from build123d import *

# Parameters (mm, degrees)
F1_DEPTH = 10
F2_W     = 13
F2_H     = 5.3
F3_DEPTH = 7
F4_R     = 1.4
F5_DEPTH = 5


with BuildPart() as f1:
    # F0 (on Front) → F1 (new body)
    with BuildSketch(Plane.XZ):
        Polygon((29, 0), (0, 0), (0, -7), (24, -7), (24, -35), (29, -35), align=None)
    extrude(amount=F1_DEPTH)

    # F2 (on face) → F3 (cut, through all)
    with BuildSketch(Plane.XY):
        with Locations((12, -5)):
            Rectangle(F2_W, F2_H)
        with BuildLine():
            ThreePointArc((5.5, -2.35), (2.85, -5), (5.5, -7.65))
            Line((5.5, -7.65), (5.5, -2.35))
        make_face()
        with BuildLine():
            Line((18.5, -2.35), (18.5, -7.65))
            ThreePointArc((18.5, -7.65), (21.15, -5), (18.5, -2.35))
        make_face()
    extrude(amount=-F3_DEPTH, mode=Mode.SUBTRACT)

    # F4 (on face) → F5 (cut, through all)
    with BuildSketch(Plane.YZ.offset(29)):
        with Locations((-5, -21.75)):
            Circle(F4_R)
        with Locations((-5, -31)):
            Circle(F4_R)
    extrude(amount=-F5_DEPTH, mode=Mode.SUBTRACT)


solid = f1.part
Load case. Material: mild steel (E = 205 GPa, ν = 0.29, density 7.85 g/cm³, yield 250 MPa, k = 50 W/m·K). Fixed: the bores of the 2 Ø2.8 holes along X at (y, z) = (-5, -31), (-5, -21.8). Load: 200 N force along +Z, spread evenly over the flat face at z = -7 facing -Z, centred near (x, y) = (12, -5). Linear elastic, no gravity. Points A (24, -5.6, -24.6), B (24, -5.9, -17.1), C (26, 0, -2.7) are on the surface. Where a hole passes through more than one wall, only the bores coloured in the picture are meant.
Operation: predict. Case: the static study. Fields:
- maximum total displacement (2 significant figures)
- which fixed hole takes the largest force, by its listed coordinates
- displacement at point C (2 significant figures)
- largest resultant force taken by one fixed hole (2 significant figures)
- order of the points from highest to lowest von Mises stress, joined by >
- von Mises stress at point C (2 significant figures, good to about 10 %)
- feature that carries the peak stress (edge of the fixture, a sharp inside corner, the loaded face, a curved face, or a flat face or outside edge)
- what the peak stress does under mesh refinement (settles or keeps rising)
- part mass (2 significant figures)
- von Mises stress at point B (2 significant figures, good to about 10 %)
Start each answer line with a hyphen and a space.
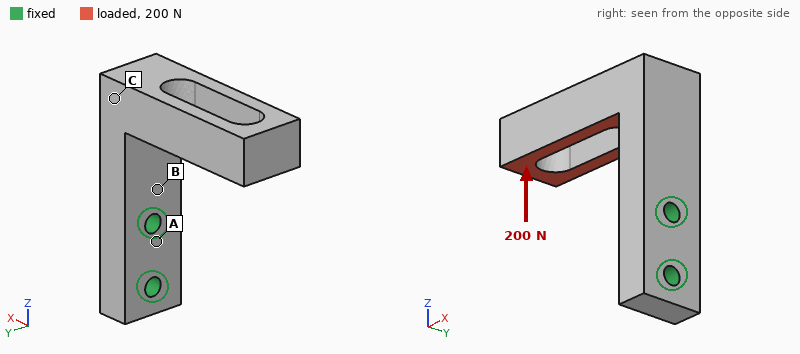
- 81 µm
- (-5, -21.8)
- 24 µm
- 190 N
- B > C > A
- 26 MPa
- edge of the fixture
- keeps rising
- 21 g
- 77 MPa
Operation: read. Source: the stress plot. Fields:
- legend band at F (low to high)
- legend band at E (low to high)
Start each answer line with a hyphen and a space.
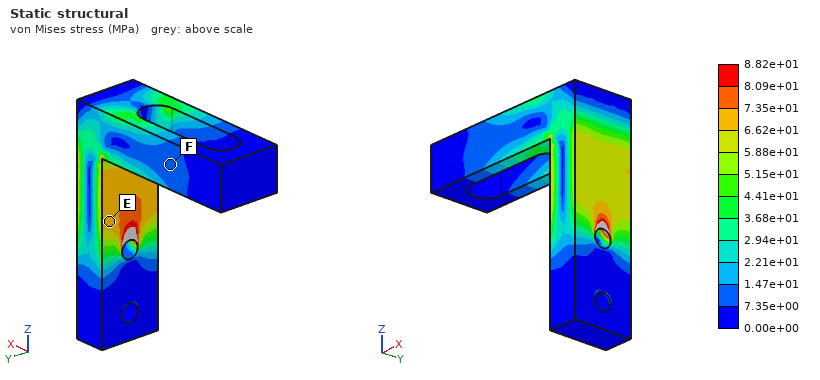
- 7.35e+00 to 1.47e+01 MPa
- 6.62e+01 to 7.35e+01 MPa
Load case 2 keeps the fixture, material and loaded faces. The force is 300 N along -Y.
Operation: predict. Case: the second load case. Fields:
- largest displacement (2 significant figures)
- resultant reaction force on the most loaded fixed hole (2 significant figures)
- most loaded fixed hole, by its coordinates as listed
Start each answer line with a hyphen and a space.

- 0.12 mm
- 550 N
- (-5, -21.8)
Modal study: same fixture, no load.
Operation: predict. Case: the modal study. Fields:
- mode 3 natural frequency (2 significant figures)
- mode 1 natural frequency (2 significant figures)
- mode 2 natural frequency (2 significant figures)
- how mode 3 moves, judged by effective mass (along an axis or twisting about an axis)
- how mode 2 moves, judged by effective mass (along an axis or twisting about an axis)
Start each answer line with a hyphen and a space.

- 8900 Hz
- 2900 Hz
- 3200 Hz
- along X
- along Y
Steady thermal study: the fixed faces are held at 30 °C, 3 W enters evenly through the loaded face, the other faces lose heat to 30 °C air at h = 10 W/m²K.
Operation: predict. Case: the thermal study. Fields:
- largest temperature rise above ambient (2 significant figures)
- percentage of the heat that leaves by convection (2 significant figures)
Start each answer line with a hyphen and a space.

- 37 K
- 11 %
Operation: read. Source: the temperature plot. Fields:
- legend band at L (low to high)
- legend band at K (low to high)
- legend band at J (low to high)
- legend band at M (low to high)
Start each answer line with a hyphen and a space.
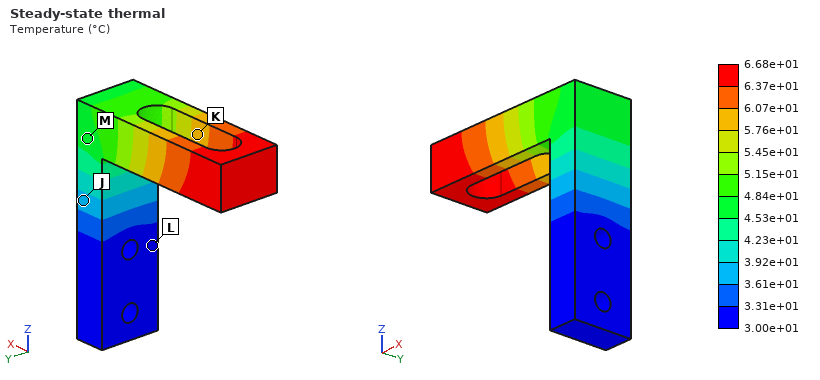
- 3.00e+01 to 3.31e+01 °C
- 5.76e+01 to 6.07e+01 °C
- 3.61e+01 to 3.92e+01 °C
- 4.53e+01 to 4.84e+01 °C
